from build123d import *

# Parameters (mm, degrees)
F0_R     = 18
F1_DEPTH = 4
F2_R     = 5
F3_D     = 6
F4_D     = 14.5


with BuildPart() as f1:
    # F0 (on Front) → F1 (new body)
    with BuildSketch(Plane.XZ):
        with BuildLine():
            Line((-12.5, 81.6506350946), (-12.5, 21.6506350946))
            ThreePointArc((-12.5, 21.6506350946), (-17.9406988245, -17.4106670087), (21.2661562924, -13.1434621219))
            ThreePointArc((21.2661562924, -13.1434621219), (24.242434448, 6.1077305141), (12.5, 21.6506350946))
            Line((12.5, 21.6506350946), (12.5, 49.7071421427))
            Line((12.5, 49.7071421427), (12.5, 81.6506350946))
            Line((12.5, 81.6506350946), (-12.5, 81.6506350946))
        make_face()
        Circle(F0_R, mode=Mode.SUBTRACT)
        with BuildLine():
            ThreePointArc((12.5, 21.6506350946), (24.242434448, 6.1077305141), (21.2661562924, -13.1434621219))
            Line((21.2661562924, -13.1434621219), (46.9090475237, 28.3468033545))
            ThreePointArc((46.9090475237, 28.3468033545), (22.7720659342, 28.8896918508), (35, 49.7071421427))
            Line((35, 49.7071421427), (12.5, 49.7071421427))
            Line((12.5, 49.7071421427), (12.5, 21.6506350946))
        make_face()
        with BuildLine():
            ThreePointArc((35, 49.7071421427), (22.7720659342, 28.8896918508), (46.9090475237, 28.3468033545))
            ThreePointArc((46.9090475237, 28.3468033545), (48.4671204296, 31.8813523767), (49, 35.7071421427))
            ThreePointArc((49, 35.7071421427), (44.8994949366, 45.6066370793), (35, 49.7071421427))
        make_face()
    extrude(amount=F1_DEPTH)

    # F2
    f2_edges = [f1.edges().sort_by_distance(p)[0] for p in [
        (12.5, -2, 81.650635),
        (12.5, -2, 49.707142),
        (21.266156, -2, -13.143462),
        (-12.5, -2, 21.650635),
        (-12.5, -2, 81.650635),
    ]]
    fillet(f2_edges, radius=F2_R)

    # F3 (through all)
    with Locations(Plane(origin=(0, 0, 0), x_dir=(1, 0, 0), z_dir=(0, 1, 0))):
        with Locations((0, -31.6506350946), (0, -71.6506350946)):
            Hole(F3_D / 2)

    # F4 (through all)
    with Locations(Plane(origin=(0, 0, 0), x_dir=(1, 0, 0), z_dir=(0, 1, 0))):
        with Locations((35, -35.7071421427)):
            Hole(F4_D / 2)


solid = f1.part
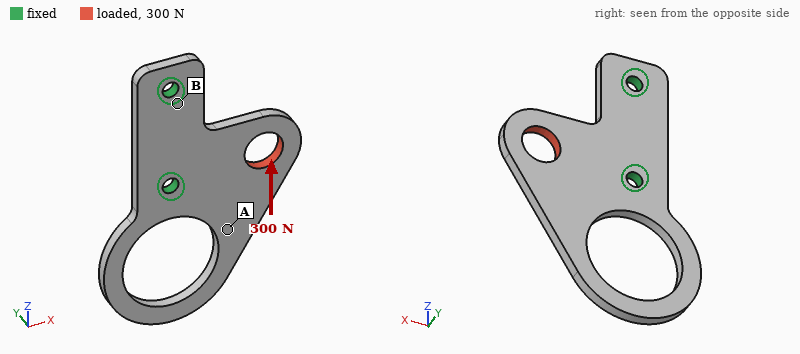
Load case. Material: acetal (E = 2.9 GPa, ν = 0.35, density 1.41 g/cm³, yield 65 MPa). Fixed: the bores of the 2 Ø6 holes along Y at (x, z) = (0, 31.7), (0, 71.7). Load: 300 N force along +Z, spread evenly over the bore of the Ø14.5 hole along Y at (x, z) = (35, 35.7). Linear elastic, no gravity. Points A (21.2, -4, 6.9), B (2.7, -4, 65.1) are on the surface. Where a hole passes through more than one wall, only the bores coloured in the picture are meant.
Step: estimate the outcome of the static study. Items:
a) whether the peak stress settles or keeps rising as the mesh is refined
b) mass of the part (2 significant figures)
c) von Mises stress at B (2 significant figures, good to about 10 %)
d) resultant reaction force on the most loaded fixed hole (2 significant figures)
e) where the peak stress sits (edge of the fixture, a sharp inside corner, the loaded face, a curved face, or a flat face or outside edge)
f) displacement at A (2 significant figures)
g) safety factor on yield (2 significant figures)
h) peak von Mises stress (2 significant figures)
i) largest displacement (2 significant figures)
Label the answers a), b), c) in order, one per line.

a) settles
b) 19 g
c) 7.2 MPa
d) 270 N
e) a curved face
f) 0.24 mm
g) 2.3
h) 28 MPa
i) 0.40 mm
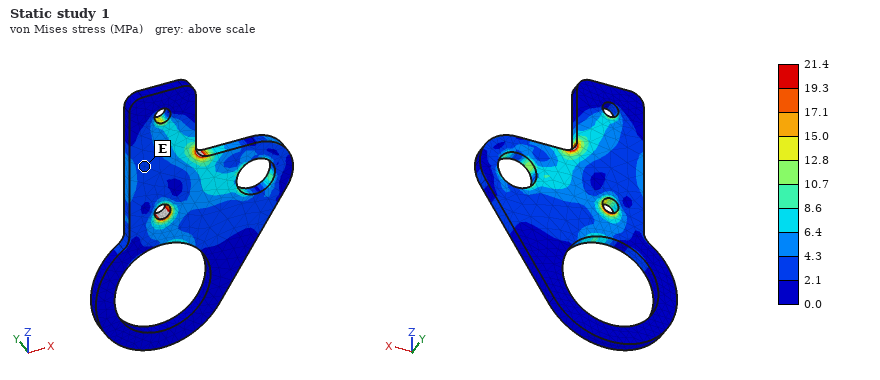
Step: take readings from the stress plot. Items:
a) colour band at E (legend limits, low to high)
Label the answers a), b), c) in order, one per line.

a) 2.1 to 4.3 MPa
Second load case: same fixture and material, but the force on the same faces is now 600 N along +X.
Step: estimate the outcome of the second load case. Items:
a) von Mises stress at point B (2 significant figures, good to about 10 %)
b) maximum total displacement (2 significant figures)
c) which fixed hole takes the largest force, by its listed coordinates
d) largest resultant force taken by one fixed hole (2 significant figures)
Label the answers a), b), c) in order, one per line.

a) 2.2 MPa
b) 0.13 mm
c) (0, 31.7)
d) 530 N
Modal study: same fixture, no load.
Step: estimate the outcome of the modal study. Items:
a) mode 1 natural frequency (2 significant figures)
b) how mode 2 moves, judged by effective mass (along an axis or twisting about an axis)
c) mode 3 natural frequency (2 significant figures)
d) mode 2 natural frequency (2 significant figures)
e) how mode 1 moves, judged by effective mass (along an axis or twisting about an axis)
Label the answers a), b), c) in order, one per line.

a) 310 Hz
b) along Y
c) 720 Hz
d) 450 Hz
e) along Y
